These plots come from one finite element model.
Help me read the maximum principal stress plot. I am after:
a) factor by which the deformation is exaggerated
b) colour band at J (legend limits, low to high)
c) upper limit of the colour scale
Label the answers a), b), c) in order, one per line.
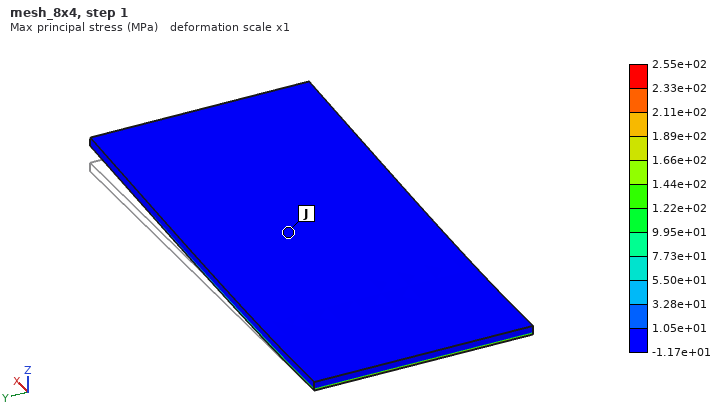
a) 1
b) -1.17e+01 to 1.05e+01 MPa
c) 2.55e+02 MPa
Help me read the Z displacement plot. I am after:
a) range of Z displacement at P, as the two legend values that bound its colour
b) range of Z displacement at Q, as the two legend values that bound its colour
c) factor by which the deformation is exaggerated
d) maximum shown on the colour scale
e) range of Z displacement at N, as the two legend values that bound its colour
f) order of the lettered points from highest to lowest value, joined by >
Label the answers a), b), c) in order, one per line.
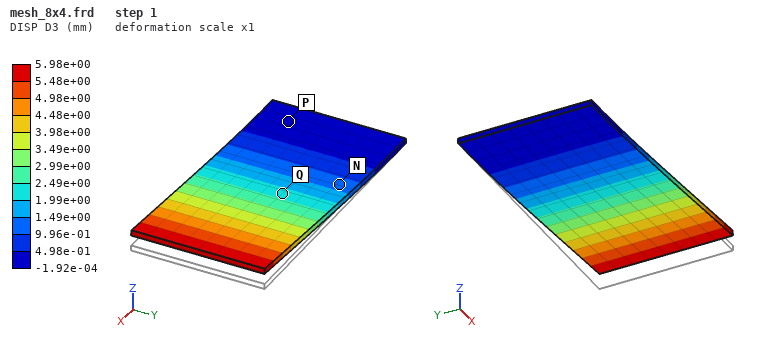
a) -1.92e-04 to 4.98e-01 mm
b) 1.99e+00 to 2.49e+00 mm
c) 1
d) 5.98e+00 mm
e) 9.96e-01 to 1.49e+00 mm
f) Q > N > P
